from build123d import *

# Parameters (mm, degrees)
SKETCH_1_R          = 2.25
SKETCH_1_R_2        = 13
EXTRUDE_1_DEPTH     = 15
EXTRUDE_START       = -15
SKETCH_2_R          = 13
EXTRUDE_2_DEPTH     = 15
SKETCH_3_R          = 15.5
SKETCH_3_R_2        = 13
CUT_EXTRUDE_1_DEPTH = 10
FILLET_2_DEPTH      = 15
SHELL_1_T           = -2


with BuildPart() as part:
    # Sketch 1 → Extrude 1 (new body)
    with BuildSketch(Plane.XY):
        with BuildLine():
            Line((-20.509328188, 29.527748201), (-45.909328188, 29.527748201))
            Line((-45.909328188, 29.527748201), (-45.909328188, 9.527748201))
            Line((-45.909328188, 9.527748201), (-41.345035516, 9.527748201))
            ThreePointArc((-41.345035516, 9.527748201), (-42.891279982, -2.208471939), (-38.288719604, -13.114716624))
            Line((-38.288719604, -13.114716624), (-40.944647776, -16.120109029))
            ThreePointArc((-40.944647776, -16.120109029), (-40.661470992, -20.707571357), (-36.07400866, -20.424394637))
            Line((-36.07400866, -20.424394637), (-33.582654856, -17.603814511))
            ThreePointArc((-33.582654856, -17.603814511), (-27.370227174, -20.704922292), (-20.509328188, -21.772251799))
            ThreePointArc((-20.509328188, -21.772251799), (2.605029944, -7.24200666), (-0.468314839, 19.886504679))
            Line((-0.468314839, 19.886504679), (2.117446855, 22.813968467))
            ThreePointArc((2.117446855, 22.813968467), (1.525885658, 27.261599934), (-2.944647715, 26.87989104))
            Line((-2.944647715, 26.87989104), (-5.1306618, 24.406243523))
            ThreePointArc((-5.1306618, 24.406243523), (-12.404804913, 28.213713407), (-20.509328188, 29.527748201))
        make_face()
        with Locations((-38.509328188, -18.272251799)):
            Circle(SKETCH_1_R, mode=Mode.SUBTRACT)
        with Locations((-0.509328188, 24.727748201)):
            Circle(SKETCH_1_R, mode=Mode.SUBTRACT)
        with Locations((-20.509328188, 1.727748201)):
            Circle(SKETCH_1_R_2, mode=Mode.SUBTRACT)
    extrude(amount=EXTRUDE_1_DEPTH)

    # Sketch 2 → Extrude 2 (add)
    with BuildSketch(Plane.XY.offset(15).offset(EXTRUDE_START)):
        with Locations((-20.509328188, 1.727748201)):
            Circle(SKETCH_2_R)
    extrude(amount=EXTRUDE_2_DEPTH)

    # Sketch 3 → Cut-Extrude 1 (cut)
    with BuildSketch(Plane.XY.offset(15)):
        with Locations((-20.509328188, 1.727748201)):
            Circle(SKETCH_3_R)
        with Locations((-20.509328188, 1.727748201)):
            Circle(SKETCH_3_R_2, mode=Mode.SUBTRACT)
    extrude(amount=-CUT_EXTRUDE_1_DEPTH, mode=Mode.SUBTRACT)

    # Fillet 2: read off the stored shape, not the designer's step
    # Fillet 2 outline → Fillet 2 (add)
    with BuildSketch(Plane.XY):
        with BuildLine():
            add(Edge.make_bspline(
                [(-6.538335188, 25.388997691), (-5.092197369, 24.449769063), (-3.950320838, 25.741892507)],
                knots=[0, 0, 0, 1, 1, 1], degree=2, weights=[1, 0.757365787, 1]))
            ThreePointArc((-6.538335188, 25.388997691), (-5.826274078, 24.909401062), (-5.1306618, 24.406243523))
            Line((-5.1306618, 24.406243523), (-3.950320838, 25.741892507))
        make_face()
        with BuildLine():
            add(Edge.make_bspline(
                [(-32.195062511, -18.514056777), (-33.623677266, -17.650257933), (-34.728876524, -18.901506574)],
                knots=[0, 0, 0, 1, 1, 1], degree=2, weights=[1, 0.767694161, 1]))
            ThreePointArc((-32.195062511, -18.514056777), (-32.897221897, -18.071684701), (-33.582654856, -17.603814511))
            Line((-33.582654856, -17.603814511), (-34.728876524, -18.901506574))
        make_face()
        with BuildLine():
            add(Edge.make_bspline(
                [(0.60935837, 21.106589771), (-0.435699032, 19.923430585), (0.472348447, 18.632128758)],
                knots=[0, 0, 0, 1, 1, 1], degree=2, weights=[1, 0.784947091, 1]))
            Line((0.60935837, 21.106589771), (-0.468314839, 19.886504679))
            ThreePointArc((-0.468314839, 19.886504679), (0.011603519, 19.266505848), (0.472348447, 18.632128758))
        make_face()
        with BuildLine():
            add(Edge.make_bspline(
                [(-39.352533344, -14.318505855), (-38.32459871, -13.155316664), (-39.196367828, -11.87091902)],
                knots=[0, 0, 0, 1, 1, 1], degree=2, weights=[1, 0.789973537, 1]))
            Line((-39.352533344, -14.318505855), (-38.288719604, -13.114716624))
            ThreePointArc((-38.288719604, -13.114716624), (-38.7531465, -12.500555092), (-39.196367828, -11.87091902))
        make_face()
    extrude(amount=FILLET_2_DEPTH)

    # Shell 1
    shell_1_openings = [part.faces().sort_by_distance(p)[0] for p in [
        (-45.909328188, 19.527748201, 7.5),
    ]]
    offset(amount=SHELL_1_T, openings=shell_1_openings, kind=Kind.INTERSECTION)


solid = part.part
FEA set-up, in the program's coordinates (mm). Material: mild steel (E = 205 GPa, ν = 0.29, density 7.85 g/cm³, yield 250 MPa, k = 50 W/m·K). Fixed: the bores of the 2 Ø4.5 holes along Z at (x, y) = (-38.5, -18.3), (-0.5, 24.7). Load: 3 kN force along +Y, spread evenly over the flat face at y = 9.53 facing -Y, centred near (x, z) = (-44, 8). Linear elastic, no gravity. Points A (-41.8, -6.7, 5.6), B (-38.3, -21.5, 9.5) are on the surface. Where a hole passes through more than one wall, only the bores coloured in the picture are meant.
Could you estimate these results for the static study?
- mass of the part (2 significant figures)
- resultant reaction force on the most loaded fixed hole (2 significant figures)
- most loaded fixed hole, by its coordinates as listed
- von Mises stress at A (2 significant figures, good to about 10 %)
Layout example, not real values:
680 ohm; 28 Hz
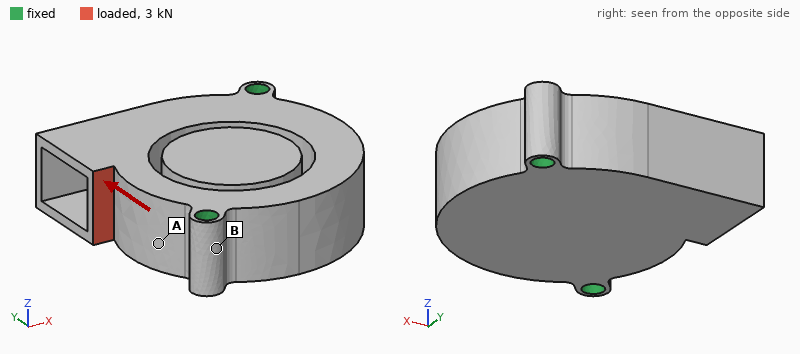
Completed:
130 g; 2.8 kN; (-38.5, -18.3); 42 MPa
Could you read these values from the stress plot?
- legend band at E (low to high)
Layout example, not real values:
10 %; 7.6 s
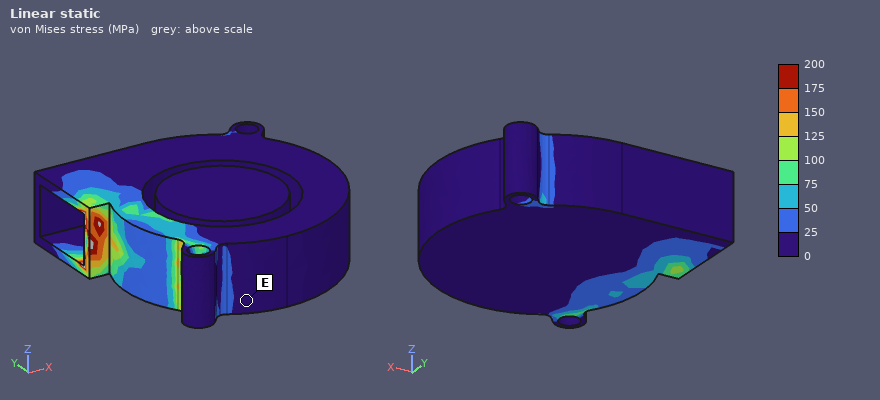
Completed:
0 to 25 MPa
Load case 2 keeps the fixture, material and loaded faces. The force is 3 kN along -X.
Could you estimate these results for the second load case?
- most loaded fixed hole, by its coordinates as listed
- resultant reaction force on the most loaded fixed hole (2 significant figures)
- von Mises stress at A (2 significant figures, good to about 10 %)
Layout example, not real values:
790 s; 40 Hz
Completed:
(-0.5, 24.7); 2.0 kN; 17 MPa
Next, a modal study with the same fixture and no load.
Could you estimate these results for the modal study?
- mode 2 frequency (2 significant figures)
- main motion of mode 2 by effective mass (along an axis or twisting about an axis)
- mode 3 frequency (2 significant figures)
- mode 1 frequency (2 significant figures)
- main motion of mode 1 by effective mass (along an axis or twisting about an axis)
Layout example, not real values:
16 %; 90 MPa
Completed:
7000 Hz; along Z; 8100 Hz; 6200 Hz; along Z
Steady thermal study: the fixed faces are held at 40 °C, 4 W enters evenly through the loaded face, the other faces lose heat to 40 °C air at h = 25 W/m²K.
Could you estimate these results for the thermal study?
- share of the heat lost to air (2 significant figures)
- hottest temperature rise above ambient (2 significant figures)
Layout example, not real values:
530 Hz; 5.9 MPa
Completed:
38 %; 22 K
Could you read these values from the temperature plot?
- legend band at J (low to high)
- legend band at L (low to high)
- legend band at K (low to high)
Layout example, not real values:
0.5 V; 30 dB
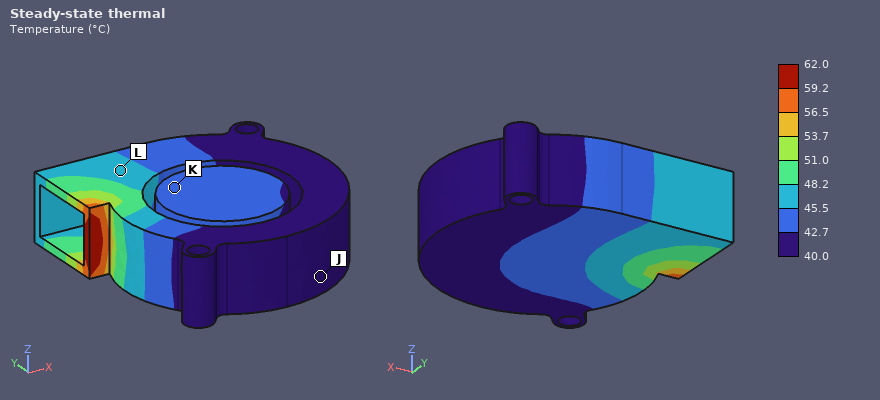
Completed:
40.0 to 42.7 °C; 45.5 to 48.2 °C; 42.7 to 45.5 °C
